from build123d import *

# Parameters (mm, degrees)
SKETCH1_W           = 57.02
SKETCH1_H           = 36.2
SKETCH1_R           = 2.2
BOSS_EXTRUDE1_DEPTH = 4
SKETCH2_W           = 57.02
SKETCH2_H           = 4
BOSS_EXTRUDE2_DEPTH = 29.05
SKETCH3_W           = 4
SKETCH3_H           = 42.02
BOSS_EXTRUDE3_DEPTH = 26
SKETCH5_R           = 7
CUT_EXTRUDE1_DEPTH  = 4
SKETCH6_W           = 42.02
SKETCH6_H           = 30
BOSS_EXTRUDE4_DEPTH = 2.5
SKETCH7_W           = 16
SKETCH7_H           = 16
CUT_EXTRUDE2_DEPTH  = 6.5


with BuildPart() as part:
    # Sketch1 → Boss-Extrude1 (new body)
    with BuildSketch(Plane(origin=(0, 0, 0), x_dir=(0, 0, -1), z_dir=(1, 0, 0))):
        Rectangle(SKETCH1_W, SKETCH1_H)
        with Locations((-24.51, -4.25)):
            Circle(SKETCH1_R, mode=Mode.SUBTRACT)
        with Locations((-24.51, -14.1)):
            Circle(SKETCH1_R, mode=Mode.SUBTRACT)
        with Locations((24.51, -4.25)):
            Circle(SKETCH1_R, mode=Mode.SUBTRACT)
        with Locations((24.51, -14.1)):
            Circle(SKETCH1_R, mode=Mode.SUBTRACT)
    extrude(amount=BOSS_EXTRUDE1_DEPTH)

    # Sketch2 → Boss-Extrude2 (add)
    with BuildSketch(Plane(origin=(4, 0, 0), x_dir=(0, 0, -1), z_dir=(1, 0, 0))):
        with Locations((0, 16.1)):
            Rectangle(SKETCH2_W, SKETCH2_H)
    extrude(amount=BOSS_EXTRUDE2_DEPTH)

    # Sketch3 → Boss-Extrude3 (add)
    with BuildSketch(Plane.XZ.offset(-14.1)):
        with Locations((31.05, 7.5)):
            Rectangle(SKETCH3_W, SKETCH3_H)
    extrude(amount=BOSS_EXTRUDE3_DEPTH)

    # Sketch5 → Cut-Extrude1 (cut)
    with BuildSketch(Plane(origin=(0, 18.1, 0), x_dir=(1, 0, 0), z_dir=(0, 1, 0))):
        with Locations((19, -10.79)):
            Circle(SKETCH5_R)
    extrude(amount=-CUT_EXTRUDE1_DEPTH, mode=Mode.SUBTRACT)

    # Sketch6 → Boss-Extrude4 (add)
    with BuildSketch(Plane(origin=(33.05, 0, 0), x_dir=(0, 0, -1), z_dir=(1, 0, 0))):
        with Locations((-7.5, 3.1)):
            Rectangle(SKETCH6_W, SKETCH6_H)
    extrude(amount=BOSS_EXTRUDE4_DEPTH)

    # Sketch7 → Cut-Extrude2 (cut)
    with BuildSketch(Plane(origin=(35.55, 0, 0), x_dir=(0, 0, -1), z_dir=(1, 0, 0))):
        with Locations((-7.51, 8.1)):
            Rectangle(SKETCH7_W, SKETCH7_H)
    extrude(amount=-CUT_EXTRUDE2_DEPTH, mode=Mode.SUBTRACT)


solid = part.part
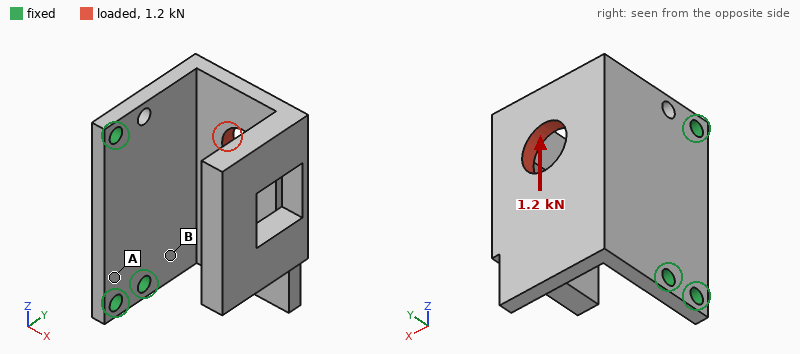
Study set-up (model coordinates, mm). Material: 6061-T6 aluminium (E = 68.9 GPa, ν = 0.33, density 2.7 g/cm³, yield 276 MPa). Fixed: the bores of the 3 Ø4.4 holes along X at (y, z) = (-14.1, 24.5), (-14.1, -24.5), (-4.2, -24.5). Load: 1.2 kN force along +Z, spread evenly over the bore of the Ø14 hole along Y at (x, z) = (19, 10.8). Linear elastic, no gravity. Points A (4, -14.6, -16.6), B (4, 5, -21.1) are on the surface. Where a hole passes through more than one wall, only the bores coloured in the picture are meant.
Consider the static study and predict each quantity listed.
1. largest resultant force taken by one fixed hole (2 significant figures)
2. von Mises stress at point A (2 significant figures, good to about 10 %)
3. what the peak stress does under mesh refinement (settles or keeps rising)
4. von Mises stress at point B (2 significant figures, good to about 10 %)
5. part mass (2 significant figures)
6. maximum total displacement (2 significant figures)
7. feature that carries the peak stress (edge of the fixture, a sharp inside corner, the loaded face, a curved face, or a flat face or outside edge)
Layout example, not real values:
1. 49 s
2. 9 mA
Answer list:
1. 870 N
2. 21 MPa
3. keeps rising
4. 77 MPa
5. 54 g
6. 0.43 mm
7. edge of the fixture
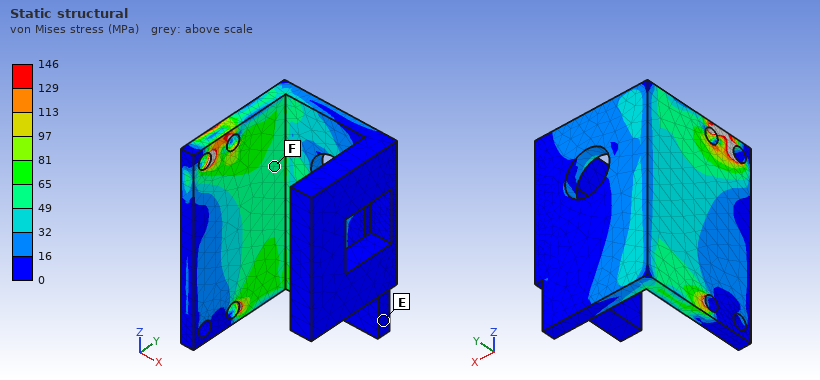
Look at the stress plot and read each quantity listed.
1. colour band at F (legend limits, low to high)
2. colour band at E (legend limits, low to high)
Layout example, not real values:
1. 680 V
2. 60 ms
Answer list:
1. 49 to 65 MPa
2. 0 to 16 MPa
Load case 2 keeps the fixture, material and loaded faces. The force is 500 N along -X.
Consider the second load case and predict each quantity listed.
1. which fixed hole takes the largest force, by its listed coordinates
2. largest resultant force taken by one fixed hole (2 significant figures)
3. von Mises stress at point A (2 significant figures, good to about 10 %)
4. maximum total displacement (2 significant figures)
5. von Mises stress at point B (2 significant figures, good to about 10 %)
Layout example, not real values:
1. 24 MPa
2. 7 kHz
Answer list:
1. (-4.2, -24.5)
2. 470 N
3. 40 MPa
4. 0.53 mm
5. 59 MPa
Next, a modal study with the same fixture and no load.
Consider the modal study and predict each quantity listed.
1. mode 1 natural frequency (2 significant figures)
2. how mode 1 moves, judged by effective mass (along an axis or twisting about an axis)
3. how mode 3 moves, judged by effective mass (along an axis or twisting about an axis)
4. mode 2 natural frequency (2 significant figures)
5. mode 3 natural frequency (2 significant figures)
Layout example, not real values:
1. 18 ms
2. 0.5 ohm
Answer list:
1. 760 Hz
2. along Y
3. along X
4. 1200 Hz
5. 1700 Hz
